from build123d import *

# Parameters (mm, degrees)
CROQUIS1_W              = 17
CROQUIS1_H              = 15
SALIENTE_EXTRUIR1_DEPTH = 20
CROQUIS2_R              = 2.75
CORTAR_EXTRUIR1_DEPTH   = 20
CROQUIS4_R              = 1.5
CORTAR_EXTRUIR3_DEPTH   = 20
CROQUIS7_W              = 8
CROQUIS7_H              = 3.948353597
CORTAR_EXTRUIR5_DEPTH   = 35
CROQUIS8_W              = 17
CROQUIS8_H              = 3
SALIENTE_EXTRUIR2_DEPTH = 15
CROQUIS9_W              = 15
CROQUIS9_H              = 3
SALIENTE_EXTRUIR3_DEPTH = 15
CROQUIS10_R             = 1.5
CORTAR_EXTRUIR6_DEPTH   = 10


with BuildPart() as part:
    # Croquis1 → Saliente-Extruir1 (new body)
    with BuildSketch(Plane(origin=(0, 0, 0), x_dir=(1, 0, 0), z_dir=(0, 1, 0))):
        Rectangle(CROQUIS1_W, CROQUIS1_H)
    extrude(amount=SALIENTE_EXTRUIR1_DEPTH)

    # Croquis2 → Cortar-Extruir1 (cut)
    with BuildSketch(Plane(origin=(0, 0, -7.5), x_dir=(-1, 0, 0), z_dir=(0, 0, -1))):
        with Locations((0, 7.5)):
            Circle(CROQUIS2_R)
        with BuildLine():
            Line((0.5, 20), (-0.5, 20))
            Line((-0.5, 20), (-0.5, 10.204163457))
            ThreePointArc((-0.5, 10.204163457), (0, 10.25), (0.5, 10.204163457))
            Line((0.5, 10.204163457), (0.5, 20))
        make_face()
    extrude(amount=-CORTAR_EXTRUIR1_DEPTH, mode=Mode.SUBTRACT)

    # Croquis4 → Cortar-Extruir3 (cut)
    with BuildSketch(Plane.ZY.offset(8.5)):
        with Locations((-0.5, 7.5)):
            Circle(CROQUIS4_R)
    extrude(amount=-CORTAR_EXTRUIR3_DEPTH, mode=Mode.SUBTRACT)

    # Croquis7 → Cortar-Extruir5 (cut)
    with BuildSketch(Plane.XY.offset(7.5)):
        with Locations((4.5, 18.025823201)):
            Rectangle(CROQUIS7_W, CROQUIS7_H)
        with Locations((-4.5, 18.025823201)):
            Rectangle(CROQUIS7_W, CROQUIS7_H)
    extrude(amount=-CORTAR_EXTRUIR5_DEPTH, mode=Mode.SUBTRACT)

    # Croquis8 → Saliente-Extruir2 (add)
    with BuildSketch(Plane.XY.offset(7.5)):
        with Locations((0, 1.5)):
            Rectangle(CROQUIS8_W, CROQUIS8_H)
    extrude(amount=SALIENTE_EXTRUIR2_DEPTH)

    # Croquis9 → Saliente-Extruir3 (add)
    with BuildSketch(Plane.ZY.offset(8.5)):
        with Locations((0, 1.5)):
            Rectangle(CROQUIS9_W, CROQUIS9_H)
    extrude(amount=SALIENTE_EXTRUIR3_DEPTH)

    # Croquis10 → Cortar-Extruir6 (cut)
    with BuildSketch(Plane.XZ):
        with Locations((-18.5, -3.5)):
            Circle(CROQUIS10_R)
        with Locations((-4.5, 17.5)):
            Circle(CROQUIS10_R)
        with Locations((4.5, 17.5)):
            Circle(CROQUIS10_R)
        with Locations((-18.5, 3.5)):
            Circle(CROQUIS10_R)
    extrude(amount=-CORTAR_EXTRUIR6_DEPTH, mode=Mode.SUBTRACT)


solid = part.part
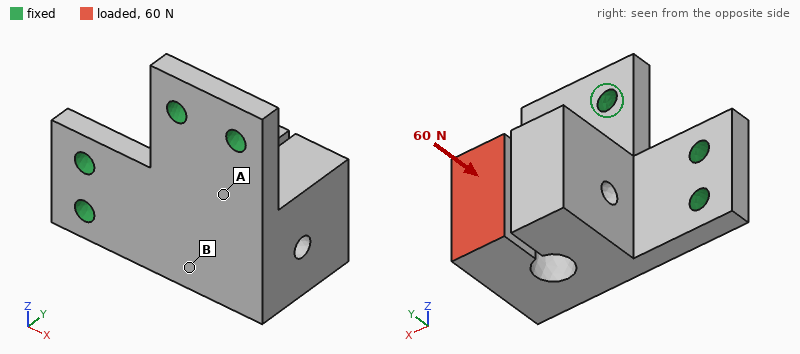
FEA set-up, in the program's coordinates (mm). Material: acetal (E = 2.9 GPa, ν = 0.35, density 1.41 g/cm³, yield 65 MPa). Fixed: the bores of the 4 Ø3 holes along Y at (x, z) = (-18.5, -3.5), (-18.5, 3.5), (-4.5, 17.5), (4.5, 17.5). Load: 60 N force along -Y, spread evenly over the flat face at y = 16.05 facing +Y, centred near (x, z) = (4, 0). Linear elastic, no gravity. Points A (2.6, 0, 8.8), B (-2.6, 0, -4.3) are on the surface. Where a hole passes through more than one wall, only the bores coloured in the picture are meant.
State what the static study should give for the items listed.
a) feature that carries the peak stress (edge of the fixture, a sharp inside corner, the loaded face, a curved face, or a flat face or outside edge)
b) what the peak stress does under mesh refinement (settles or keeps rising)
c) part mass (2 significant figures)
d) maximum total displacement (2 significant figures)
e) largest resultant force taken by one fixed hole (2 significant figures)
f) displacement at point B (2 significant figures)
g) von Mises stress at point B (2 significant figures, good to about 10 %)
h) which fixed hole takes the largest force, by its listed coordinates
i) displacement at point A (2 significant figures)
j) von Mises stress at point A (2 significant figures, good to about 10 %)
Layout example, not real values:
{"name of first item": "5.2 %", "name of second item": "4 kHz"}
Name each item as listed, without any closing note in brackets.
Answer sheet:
{"feature that carries the peak stress": "edge of the fixture", "what the peak stress does under mesh refinement": "keeps rising", "part mass": "6.9 g", "maximum total displacement": "0.56 mm", "largest resultant force taken by one fixed hole": "54 N", "displacement at point B": "0.23 mm", "von Mises stress at point B": "3.4 MPa", "which fixed hole takes the largest force, by its listed coordinates": "(4.5, 17.5)", "displacement at point A": "0.11 mm", "von Mises stress at point A": "6.8 MPa"}
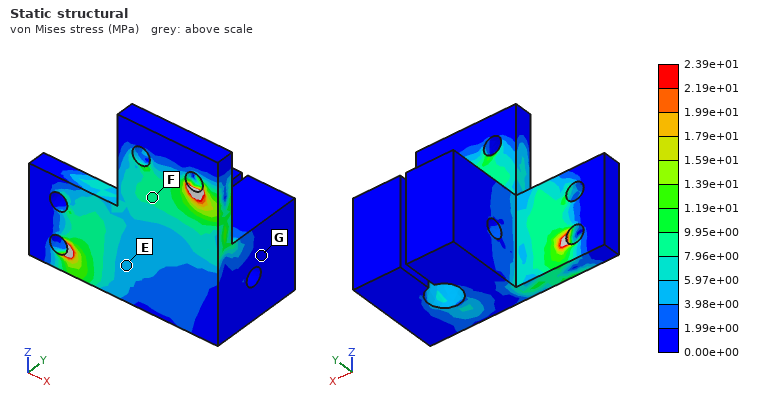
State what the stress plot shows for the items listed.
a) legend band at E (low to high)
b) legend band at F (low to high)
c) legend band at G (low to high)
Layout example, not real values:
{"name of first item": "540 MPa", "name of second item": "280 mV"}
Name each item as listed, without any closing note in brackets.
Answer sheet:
{"legend band at E": "3.98e+00 to 5.97e+00 MPa", "legend band at F": "7.96e+00 to 9.95e+00 MPa", "legend band at G": "0.00e+00 to 1.99e+00 MPa"}
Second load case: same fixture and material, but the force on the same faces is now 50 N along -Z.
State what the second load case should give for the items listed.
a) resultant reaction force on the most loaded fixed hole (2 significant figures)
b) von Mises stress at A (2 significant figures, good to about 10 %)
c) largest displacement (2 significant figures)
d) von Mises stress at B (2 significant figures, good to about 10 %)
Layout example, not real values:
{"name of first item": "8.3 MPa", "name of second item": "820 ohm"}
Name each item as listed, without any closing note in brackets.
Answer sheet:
{"resultant reaction force on the most loaded fixed hole": "46 N", "von Mises stress at A": "7.5 MPa", "largest displacement": "0.49 mm", "von Mises stress at B": "4.4 MPa"}
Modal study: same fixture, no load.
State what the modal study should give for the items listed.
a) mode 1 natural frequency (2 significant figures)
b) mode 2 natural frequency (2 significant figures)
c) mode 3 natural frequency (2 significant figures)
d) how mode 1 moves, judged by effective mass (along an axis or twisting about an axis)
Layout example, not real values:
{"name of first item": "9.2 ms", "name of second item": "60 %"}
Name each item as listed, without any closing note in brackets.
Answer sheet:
{"mode 1 natural frequency": "990 Hz", "mode 2 natural frequency": "2600 Hz", "mode 3 natural frequency": "3600 Hz", "how mode 1 moves, judged by effective mass": "along Y"}
